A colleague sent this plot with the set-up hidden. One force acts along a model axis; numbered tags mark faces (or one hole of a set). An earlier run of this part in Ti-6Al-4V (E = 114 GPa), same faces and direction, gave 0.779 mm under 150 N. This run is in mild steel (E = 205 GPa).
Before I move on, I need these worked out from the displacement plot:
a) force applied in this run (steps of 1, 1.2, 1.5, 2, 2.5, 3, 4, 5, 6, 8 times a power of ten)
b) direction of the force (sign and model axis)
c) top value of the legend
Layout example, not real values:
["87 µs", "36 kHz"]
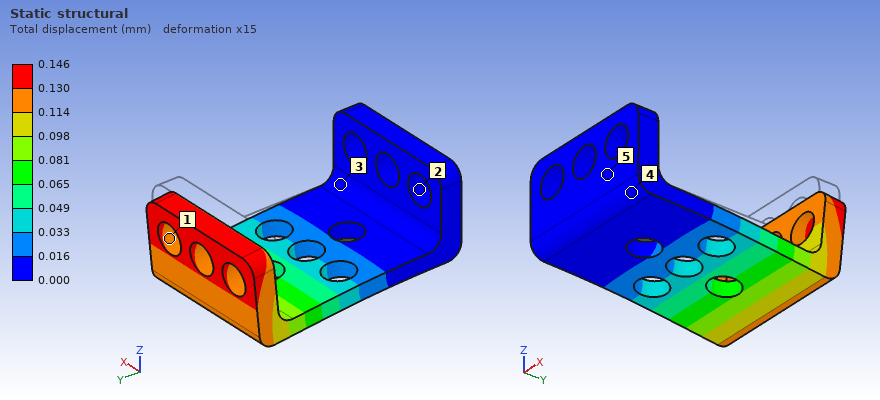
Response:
["50 N", "-Z", "0.146 mm"]
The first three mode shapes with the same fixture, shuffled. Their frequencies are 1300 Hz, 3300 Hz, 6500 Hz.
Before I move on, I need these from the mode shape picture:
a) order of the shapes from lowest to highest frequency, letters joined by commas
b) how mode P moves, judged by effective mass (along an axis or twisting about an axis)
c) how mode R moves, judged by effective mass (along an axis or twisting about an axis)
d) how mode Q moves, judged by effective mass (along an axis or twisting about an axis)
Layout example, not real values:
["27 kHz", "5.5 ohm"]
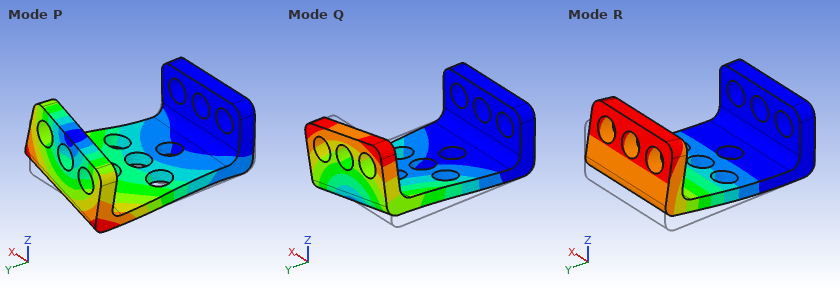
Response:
["R, Q, P", "along X", "along Z", "along X"]
